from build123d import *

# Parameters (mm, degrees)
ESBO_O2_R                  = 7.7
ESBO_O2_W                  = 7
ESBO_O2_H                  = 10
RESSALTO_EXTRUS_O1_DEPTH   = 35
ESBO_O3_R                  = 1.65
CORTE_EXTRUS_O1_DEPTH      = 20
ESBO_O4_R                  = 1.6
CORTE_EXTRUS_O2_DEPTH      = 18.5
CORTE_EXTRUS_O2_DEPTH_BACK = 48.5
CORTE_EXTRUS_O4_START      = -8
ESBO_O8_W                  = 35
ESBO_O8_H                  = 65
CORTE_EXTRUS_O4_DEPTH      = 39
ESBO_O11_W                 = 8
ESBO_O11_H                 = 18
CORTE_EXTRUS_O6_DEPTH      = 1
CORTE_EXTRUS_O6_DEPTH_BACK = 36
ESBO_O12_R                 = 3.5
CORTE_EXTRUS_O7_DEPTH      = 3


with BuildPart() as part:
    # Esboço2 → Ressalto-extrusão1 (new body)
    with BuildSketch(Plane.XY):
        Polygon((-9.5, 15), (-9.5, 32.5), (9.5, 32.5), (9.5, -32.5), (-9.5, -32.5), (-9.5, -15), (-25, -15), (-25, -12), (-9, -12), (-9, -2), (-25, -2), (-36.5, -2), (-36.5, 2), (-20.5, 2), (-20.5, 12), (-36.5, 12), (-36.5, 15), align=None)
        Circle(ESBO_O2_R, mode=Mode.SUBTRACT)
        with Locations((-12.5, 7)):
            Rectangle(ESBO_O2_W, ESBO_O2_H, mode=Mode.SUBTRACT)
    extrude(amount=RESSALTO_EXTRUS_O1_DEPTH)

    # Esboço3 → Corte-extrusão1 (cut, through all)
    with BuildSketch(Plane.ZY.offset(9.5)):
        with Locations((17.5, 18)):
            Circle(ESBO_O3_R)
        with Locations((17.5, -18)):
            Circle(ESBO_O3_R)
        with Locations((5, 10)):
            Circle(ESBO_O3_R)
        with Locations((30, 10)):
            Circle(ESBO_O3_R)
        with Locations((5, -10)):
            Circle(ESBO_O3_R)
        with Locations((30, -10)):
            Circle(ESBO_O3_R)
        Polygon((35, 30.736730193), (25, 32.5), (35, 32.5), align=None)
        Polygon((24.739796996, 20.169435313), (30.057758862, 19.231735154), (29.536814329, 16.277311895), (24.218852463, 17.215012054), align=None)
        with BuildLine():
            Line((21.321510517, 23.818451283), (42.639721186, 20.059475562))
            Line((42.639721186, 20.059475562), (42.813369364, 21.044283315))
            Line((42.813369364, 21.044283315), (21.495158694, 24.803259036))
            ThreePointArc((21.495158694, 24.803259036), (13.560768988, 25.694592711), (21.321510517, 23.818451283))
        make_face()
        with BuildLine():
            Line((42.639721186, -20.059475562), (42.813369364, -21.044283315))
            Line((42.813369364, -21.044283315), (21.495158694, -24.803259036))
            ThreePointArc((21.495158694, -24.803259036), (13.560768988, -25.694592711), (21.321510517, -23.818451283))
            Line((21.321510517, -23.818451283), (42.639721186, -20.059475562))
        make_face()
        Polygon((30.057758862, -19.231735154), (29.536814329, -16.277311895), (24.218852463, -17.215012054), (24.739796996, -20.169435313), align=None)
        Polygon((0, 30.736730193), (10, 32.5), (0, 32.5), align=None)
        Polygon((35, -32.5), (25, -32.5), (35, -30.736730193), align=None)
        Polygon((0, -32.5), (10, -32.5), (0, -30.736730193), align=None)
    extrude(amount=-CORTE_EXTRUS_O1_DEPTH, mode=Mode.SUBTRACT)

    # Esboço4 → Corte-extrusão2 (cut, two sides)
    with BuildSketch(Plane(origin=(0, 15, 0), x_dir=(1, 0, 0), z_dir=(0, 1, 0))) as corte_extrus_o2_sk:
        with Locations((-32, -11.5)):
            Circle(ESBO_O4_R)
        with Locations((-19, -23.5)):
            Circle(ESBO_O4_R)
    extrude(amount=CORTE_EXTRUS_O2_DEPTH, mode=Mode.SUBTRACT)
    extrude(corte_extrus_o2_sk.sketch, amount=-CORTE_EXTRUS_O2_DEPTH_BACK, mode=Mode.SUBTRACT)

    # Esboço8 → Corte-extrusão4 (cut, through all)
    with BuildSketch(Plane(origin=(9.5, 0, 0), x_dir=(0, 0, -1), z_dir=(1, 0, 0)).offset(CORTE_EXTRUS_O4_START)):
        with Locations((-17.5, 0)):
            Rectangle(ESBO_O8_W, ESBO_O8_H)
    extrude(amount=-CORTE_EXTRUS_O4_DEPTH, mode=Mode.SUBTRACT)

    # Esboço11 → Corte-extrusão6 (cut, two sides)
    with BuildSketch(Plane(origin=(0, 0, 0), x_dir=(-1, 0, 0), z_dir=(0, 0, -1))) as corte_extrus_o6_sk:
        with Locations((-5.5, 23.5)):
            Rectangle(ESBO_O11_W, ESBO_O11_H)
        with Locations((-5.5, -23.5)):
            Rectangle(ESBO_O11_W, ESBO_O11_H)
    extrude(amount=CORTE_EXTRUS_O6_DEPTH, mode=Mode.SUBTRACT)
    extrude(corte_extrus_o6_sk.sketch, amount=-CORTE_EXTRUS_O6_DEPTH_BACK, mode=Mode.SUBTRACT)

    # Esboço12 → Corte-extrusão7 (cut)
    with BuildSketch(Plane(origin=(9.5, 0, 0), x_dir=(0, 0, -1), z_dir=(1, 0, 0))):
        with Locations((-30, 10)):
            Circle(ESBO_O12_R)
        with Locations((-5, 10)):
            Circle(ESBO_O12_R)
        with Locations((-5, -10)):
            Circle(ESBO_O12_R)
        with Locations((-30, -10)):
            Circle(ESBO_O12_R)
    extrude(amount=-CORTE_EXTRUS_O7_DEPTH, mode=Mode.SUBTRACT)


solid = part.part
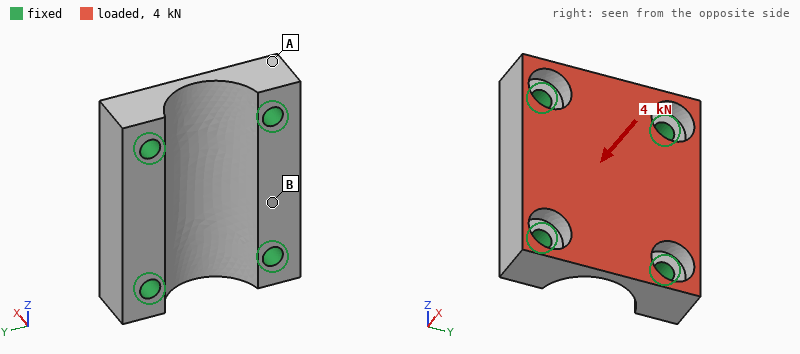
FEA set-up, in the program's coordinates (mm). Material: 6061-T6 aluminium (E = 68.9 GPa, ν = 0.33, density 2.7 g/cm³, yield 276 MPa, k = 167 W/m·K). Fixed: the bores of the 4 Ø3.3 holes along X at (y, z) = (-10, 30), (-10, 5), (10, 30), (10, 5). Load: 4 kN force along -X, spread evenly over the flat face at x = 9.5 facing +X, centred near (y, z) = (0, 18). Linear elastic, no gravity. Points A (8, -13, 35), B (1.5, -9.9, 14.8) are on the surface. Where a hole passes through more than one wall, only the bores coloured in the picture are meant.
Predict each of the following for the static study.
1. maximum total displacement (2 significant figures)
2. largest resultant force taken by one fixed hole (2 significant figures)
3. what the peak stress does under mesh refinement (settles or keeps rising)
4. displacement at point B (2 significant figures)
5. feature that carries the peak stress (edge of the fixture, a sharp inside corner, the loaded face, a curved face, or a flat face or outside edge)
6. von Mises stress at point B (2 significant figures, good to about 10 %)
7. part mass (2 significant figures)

13 µm
1.2 kN
keeps rising
6.8 µm
edge of the fixture
17 MPa
14 g
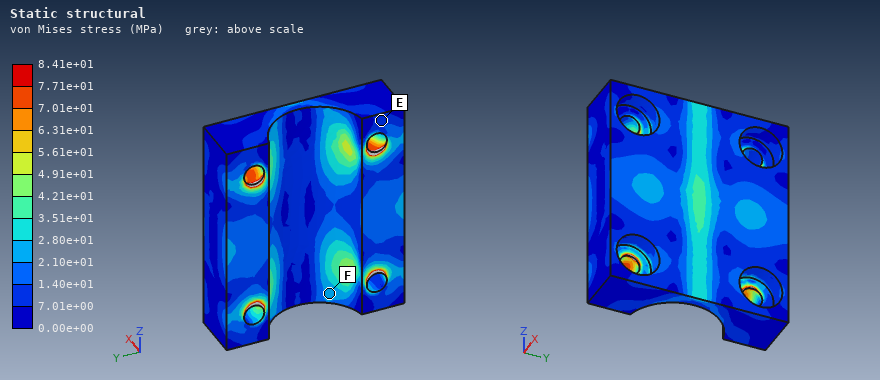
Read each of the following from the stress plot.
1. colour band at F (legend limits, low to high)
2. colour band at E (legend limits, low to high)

2.10e+01 to 2.80e+01 MPa
7.01e+00 to 1.40e+01 MPa
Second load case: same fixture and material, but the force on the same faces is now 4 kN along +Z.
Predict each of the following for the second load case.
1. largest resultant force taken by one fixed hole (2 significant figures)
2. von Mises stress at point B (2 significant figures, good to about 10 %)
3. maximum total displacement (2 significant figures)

1.1 kN
6.5 MPa
8.4 µm
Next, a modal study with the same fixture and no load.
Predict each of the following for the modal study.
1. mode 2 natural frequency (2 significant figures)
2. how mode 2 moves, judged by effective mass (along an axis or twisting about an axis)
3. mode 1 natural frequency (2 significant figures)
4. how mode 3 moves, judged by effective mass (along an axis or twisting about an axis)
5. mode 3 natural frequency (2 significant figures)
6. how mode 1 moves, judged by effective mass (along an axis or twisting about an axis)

38 kHz
along Y
36 kHz
along Y
41 kHz
along X
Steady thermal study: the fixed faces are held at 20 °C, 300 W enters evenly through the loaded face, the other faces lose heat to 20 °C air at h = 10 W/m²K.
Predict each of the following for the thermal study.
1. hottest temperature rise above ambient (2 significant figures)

61 K
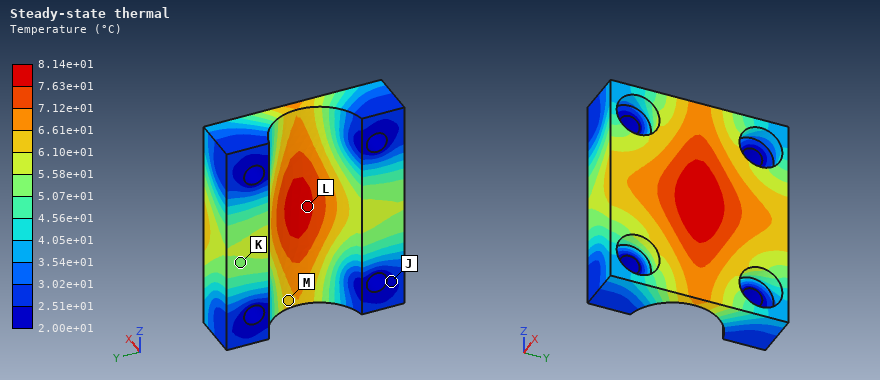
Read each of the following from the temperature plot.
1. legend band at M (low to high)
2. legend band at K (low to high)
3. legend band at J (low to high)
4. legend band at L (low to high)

6.10e+01 to 6.61e+01 °C
5.07e+01 to 5.58e+01 °C
2.00e+01 to 2.51e+01 °C
7.63e+01 to 8.14e+01 °C
